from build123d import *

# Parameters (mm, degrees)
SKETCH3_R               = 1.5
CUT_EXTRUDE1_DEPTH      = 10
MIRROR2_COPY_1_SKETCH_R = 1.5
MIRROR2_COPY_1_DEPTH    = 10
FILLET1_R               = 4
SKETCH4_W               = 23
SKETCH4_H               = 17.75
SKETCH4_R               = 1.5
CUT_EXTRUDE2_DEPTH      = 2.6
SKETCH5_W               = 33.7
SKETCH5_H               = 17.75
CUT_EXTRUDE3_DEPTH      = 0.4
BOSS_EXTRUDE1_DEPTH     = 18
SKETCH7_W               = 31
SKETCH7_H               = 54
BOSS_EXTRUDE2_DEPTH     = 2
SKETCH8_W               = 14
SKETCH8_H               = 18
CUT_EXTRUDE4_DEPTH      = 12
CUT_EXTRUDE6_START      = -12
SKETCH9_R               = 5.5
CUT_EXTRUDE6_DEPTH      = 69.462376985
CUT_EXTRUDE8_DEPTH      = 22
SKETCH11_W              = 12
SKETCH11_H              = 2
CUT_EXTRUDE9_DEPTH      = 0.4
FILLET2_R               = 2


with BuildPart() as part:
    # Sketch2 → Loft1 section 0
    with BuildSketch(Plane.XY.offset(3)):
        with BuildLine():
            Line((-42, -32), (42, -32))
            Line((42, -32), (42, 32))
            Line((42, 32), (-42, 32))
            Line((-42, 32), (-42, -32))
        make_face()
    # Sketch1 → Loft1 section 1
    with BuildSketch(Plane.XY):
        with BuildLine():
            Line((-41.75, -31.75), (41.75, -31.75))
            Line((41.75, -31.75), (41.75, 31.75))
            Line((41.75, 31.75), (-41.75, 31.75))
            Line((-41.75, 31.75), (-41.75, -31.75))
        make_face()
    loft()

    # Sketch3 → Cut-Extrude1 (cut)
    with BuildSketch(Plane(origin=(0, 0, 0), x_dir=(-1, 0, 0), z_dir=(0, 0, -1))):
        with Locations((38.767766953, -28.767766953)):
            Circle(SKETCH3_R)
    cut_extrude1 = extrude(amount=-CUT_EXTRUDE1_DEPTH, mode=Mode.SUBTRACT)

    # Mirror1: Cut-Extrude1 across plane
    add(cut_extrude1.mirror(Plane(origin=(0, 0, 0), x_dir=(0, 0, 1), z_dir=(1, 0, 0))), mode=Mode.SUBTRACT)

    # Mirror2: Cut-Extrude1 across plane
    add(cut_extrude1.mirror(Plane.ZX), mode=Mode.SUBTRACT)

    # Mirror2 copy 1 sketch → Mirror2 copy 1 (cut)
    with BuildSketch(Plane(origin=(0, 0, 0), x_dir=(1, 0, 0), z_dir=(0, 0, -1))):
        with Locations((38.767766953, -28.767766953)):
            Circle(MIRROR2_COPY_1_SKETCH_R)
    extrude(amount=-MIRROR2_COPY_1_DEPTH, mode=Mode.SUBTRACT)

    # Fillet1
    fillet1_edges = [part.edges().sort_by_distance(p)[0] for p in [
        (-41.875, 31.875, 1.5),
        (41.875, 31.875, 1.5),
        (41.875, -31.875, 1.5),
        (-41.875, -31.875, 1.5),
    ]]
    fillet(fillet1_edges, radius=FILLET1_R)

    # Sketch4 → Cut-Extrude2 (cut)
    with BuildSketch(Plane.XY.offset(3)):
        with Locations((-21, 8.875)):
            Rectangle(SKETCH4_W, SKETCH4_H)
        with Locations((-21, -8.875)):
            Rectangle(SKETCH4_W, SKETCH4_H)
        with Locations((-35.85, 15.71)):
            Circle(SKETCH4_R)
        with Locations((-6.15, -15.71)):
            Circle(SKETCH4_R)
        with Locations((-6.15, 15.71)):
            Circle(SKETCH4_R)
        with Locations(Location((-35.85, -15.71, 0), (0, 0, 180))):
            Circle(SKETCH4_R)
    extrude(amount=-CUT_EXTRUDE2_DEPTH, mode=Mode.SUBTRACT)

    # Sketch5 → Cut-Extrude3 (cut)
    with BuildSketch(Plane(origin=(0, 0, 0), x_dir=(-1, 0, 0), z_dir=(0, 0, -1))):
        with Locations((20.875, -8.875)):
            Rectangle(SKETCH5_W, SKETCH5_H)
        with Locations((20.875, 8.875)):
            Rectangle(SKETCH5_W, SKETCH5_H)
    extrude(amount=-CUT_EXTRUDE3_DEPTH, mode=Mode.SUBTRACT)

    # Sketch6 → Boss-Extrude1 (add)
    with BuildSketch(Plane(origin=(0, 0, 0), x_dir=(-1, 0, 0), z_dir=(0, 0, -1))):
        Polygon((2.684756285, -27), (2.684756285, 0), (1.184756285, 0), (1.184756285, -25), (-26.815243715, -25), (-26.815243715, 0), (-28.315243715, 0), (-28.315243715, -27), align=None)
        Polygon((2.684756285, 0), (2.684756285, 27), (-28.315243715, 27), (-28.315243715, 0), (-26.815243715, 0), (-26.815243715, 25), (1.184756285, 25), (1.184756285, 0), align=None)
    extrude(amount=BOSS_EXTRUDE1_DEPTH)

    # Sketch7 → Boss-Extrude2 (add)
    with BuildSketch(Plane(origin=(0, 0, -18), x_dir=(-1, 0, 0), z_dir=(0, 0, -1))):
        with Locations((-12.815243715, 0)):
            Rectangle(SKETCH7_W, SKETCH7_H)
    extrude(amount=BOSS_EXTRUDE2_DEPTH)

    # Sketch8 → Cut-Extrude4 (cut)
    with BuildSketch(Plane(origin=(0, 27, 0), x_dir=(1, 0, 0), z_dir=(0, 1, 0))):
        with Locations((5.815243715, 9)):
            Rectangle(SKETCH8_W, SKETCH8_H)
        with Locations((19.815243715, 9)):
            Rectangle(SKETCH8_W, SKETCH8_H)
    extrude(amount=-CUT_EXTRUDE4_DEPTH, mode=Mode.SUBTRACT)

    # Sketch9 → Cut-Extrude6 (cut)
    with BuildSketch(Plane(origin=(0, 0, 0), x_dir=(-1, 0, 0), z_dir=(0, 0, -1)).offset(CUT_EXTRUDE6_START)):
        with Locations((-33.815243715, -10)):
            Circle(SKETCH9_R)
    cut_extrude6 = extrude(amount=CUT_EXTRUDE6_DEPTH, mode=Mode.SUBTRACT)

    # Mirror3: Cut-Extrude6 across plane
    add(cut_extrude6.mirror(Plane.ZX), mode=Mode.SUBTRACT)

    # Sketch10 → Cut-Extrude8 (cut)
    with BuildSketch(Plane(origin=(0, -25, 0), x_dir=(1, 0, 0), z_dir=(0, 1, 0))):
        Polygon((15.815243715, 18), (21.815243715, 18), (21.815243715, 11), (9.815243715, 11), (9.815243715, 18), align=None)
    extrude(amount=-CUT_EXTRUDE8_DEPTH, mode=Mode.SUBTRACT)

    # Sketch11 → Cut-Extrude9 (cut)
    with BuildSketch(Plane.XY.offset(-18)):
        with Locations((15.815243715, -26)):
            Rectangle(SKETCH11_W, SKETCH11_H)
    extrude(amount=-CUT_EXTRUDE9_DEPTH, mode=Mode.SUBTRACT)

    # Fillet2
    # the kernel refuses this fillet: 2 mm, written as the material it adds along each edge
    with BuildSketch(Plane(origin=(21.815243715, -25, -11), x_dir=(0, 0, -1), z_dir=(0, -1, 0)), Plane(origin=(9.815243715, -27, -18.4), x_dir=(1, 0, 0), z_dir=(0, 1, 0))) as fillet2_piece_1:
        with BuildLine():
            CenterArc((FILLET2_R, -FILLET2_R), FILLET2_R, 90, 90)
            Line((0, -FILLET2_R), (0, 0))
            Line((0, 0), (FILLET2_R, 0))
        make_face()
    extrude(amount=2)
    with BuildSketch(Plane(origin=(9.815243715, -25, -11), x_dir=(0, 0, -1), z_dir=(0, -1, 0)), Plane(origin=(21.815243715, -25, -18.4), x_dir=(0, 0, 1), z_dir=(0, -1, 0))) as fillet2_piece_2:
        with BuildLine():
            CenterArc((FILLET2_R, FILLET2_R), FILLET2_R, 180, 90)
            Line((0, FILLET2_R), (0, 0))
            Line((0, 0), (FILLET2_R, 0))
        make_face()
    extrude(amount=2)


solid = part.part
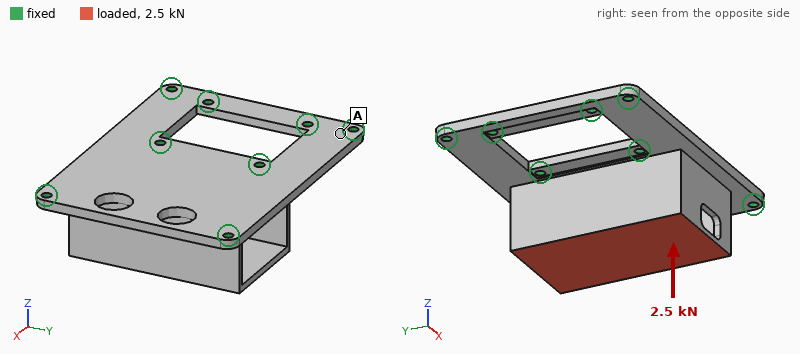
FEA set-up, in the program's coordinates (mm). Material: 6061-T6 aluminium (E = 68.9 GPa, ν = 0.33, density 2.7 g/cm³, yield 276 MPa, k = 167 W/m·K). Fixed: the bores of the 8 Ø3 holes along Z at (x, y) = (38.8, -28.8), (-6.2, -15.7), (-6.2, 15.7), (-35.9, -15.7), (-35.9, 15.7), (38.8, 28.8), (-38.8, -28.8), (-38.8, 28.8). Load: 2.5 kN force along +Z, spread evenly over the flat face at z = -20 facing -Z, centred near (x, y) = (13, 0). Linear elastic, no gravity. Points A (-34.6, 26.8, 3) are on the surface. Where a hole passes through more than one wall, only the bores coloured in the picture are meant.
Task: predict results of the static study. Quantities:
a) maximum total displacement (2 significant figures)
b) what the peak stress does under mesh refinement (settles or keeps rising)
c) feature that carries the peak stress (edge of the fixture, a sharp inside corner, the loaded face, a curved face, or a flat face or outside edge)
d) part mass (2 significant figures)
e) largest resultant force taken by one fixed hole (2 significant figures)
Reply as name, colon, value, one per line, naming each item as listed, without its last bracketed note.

maximum total displacement: 0.21 mm
what the peak stress does under mesh refinement: keeps rising
feature that carries the peak stress: edge of the fixture
part mass: 53 g
largest resultant force taken by one fixed hole: 740 N
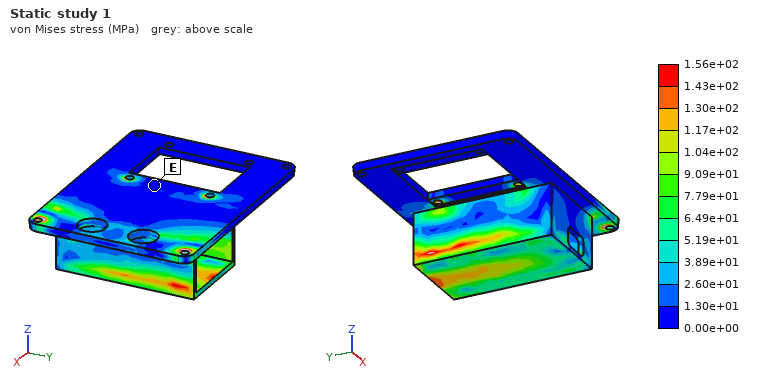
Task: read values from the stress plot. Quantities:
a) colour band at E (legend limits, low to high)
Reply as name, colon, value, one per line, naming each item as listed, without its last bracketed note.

colour band at E: 0.00e+00 to 1.30e+01 MPa
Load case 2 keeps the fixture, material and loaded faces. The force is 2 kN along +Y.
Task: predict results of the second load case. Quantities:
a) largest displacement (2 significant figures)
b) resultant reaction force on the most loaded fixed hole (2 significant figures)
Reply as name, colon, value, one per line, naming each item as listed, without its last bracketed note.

largest displacement: 74 µm
resultant reaction force on the most loaded fixed hole: 1.0 kN
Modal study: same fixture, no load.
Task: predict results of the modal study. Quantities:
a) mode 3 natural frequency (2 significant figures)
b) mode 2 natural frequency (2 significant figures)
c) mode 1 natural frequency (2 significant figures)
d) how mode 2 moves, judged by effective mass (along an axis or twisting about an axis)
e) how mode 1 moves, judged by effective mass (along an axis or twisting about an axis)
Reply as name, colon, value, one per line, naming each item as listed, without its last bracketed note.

mode 3 natural frequency: 6600 Hz
mode 2 natural frequency: 5100 Hz
mode 1 natural frequency: 3900 Hz
how mode 2 moves, judged by effective mass: along Z
how mode 1 moves, judged by effective mass: along X
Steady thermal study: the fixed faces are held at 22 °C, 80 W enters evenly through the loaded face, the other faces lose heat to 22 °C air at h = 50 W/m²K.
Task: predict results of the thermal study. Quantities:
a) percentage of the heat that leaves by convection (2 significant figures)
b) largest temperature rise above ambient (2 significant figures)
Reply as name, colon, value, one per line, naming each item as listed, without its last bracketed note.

percentage of the heat that leaves by convection: 25 %
largest temperature rise above ambient: 74 K
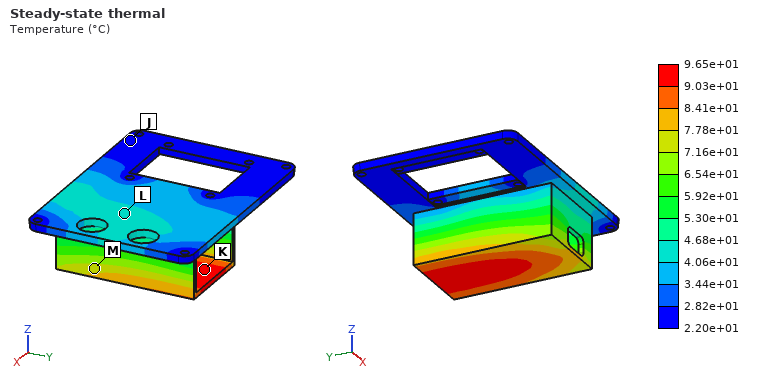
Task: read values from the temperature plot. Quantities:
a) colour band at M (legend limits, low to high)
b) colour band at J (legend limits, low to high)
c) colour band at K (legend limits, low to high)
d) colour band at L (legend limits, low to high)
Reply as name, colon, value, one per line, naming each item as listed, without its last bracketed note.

colour band at M: 7.16e+01 to 7.78e+01 °C
colour band at J: 2.20e+01 to 2.82e+01 °C
colour band at K: 9.03e+01 to 9.65e+01 °C
colour band at L: 4.06e+01 to 4.68e+01 °C
